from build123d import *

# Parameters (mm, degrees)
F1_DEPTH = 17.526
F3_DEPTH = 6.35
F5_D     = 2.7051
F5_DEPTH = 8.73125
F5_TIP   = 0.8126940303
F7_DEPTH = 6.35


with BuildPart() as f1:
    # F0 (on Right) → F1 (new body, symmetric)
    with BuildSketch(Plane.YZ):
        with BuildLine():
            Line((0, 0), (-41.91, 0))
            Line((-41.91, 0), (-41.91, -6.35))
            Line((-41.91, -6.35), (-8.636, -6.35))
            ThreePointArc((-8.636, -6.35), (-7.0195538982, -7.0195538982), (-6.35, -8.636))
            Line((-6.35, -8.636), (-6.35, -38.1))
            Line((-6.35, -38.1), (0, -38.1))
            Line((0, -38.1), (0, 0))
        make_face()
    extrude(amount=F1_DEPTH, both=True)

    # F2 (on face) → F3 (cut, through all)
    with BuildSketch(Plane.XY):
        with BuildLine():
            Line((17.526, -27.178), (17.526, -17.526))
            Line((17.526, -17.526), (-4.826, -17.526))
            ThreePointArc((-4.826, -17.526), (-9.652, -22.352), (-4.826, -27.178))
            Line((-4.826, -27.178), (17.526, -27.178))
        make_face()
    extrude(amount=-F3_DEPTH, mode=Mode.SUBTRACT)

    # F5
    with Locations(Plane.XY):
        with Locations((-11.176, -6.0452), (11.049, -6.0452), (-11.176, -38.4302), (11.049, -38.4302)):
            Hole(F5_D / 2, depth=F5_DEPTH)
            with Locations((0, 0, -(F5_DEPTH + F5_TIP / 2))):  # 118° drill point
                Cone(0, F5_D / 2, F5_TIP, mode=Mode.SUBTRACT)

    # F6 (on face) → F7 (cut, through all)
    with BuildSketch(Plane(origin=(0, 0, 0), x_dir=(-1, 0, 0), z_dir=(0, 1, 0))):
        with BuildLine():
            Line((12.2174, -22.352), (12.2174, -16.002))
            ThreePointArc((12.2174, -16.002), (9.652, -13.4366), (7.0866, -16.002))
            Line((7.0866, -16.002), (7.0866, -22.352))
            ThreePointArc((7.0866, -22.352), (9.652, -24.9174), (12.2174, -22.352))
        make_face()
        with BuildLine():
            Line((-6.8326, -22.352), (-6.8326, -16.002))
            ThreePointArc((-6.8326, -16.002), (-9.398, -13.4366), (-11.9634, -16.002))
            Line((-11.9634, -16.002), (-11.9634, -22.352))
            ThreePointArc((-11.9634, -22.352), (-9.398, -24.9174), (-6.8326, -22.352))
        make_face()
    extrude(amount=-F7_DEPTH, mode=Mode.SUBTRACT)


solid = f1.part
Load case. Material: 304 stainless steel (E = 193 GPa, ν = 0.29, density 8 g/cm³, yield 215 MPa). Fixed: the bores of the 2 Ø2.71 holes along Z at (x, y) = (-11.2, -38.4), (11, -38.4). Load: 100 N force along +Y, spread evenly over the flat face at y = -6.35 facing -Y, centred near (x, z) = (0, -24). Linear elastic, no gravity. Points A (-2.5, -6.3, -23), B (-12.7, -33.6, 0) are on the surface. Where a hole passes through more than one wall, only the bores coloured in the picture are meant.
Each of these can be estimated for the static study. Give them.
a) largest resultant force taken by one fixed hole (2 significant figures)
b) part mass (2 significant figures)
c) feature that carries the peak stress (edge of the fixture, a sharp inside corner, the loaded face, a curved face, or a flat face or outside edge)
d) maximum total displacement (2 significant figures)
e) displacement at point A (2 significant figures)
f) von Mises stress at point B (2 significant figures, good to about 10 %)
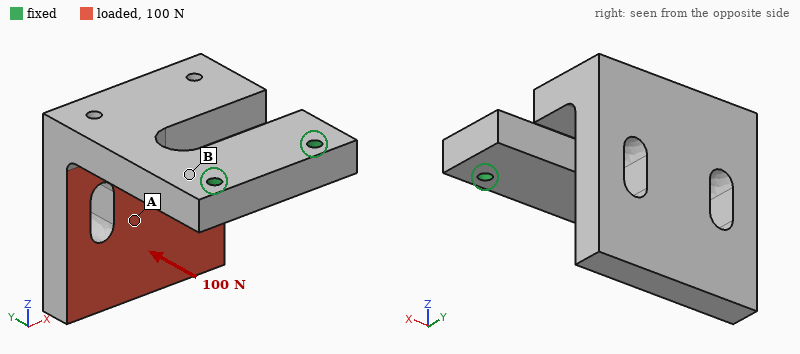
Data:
73 N
110 g
a curved face
77 µm
43 µm
23 MPa
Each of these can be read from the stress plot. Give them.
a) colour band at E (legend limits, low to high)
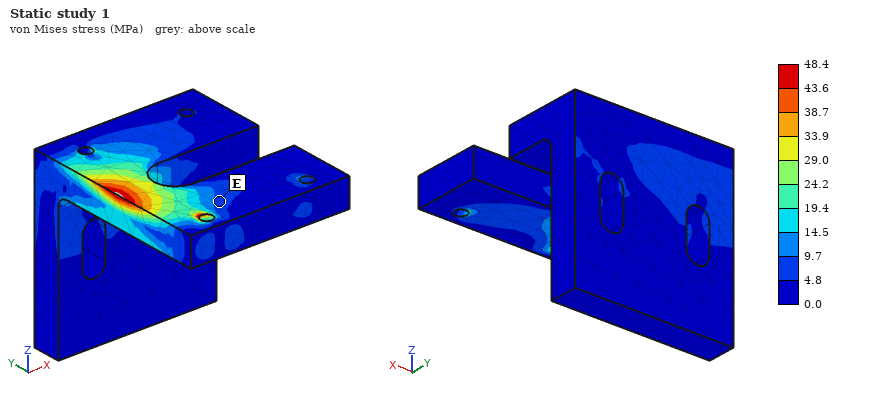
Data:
4.8 to 9.7 MPa
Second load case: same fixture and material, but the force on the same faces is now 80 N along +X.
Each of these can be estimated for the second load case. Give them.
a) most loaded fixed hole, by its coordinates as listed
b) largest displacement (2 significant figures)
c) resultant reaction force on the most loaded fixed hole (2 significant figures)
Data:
(11, -38.4)
59 µm
160 N
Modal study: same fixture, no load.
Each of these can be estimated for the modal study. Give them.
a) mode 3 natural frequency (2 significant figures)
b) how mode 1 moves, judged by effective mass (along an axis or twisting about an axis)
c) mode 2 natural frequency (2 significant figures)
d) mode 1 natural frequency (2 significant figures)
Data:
2000 Hz
along Z
950 Hz
730 Hz
